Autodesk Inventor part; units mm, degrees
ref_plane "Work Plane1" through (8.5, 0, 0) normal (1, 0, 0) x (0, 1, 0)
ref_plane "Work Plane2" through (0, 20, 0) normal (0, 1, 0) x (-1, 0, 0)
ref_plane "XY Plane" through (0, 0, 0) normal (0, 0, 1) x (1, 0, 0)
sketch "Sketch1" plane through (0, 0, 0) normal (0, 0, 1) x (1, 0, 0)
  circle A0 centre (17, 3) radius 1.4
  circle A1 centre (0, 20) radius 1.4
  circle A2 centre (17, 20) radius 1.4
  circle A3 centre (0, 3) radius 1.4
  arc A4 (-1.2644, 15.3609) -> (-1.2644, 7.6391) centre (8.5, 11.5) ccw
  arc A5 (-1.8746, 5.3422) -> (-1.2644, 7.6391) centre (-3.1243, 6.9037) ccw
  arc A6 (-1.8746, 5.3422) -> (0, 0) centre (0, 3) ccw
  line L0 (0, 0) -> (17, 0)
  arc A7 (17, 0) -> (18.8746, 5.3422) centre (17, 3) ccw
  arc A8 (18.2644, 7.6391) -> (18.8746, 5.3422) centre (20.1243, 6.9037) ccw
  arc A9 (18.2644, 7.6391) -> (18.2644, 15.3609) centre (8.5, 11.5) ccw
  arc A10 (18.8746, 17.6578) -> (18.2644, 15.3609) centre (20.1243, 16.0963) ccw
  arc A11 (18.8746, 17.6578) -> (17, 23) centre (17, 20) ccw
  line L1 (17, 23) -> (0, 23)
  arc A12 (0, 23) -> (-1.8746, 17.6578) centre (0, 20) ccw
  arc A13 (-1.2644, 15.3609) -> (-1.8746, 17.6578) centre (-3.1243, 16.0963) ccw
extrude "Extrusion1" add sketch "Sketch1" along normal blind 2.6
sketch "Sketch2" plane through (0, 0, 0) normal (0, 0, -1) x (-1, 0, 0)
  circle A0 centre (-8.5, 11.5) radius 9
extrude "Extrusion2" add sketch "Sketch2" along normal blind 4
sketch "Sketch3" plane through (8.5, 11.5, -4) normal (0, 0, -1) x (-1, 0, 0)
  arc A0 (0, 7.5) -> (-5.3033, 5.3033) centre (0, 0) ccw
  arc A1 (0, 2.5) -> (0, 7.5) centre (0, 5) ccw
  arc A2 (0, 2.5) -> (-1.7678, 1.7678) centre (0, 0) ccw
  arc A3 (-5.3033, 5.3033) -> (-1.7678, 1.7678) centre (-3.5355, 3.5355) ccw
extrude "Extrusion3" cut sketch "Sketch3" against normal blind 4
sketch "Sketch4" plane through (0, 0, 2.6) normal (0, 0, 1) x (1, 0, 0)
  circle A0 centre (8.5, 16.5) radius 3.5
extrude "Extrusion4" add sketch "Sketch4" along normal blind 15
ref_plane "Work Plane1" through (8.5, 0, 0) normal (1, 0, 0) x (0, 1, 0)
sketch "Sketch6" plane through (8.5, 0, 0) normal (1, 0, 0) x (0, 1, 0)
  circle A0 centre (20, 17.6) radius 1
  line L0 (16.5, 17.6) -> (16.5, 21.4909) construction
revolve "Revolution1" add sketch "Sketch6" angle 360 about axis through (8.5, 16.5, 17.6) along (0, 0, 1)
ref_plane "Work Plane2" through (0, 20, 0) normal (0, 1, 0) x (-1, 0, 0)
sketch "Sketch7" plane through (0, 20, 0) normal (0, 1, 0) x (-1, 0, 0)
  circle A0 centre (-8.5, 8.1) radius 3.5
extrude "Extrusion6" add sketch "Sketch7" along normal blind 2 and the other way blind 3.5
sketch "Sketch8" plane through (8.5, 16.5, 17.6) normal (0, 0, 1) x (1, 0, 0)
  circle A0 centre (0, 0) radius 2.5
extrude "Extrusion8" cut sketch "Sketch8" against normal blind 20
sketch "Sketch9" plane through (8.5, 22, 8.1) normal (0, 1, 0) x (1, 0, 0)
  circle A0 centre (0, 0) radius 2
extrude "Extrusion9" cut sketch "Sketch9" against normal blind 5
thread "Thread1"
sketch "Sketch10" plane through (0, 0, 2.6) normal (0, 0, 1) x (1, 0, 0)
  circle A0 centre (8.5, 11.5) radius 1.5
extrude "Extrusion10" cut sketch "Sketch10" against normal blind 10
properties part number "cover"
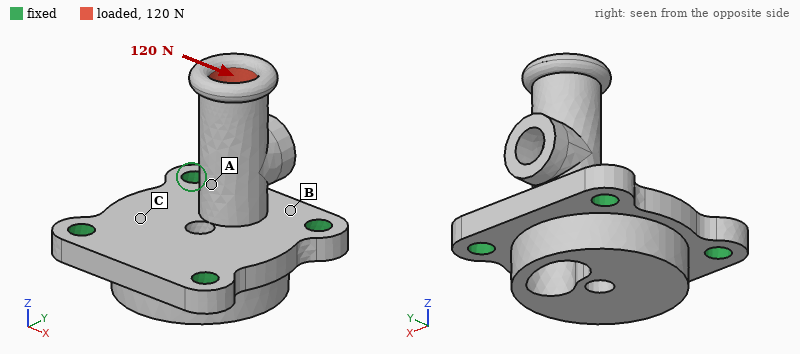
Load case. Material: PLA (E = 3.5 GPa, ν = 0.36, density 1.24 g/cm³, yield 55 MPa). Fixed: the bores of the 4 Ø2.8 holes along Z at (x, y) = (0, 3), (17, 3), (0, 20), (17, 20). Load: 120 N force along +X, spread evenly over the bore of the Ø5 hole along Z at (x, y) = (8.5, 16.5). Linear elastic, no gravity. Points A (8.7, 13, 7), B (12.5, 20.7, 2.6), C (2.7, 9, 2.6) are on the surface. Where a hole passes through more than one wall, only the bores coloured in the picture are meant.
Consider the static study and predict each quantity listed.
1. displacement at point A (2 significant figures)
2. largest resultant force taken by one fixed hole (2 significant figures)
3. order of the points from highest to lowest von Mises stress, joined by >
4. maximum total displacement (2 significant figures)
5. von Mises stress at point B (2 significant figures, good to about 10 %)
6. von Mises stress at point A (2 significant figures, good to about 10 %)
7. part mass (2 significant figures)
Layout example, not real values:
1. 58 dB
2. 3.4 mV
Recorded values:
1. 0.092 mm
2. 74 N
3. A > B > C
4. 0.36 mm
5. 6.3 MPa
6. 14 MPa
7. 2.9 g
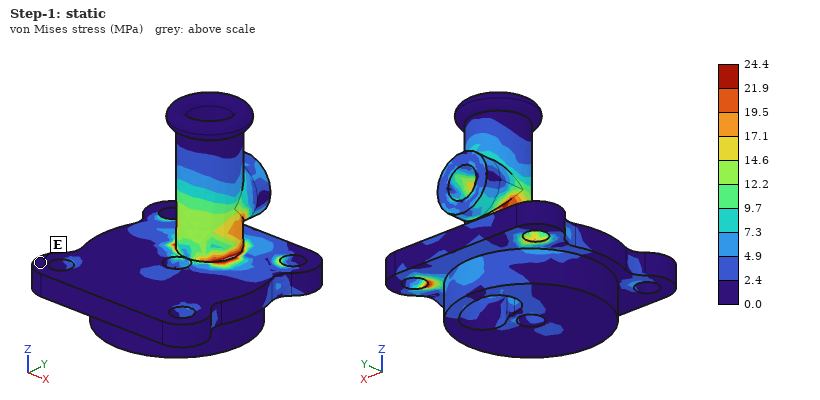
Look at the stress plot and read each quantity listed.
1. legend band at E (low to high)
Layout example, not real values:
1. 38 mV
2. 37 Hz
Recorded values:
1. 0.0 to 2.4 MPa
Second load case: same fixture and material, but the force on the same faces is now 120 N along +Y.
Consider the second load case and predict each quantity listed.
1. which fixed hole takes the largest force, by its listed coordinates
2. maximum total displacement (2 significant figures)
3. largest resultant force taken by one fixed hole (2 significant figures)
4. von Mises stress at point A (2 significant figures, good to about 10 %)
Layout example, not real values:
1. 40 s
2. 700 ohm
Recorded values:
1. (0, 20)
2. 0.41 mm
3. 58 N
4. 15 MPa
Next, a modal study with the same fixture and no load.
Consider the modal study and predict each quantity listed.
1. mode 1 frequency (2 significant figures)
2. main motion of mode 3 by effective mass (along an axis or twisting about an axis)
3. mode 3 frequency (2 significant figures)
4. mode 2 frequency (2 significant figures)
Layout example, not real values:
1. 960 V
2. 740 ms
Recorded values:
1. 4000 Hz
2. along Z
3. 10 kHz
4. 4300 Hz
